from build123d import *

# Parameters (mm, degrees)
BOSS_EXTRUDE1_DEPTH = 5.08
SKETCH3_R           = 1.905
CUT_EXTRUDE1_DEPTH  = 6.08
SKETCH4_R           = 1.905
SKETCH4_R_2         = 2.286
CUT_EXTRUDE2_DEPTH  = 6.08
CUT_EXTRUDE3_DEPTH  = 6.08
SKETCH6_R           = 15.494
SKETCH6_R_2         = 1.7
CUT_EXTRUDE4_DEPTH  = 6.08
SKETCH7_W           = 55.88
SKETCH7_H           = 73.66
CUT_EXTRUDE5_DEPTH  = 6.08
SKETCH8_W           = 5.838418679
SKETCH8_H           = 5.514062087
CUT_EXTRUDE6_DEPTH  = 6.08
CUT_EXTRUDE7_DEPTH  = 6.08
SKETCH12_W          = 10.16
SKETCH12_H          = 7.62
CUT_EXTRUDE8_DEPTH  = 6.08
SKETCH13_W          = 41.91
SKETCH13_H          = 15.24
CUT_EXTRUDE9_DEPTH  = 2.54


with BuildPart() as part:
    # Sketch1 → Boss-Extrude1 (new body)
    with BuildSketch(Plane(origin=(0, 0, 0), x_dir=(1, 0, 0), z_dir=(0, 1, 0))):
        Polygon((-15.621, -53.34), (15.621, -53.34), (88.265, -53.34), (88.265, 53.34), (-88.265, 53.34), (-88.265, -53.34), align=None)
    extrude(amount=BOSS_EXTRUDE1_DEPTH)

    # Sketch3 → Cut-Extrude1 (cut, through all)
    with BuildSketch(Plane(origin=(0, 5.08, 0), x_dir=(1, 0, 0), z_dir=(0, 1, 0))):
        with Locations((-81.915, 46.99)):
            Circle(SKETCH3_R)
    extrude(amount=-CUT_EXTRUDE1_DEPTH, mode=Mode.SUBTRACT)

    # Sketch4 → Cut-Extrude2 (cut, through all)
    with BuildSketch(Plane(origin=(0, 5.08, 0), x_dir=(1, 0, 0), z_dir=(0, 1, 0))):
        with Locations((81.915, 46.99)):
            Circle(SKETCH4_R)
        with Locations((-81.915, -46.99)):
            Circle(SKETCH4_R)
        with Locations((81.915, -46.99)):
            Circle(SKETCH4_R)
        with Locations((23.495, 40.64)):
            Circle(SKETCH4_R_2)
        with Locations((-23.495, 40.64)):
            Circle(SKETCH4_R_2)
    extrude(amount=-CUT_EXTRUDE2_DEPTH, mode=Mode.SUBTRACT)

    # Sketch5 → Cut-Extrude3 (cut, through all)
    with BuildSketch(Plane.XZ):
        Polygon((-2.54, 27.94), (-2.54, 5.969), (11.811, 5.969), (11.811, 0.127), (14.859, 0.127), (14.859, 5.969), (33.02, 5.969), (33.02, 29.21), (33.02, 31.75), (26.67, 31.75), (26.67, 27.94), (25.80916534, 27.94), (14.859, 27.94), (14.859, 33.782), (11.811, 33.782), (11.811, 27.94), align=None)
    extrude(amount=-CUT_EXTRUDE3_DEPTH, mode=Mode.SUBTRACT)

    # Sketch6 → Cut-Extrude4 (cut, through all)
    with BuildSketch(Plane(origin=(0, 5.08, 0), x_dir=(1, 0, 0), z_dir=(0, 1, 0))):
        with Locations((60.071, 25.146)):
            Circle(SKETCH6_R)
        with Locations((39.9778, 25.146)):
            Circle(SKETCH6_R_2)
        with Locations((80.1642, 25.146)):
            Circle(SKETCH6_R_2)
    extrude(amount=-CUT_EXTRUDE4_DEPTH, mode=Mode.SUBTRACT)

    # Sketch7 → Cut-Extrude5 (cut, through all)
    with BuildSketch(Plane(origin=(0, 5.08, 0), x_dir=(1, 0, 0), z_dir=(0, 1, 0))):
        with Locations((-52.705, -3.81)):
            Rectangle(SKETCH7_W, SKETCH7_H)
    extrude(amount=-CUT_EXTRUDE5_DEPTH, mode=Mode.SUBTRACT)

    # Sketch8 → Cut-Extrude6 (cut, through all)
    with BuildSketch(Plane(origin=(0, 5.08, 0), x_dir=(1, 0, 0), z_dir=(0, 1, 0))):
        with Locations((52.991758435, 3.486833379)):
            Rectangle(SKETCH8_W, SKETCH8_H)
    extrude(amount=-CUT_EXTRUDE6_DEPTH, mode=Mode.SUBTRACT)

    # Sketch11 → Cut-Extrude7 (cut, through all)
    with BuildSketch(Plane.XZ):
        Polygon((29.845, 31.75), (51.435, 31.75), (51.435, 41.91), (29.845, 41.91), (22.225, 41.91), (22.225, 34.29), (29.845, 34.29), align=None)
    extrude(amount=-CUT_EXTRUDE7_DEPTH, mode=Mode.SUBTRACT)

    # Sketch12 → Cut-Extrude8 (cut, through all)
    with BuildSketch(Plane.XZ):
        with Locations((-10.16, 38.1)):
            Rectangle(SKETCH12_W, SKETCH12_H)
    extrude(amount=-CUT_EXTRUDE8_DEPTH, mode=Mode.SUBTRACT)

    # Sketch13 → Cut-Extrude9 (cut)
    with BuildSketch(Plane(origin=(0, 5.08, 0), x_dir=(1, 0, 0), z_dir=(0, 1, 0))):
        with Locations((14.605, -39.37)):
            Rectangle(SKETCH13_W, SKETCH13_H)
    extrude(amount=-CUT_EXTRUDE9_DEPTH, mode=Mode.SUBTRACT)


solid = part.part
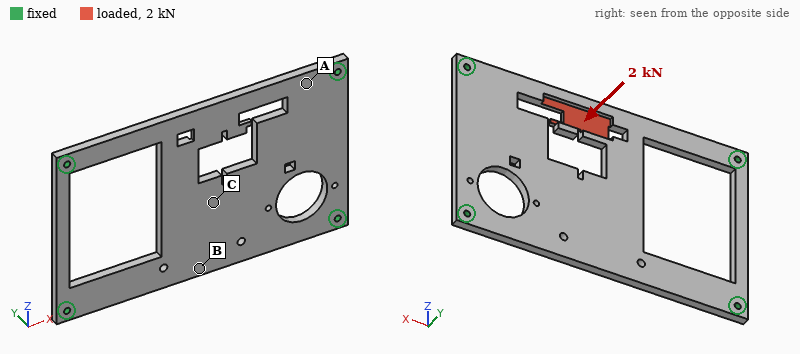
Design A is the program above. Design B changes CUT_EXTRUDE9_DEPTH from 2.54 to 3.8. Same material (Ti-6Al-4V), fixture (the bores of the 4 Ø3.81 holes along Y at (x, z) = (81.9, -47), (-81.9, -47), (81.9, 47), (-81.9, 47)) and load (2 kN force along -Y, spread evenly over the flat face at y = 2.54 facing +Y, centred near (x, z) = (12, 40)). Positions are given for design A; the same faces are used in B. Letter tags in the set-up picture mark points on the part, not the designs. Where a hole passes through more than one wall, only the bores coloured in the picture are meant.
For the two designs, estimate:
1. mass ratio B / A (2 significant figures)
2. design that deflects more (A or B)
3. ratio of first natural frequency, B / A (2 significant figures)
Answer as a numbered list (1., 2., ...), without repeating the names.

1. 0.99
2. B
3. 1.0
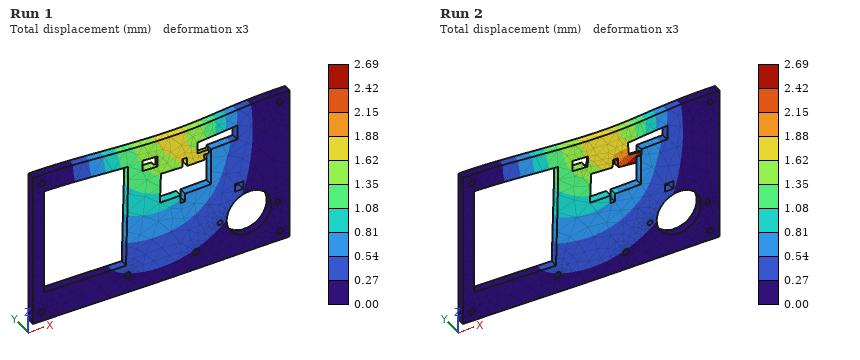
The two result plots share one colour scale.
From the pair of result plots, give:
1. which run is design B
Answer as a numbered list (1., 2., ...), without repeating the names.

1. Run 2
